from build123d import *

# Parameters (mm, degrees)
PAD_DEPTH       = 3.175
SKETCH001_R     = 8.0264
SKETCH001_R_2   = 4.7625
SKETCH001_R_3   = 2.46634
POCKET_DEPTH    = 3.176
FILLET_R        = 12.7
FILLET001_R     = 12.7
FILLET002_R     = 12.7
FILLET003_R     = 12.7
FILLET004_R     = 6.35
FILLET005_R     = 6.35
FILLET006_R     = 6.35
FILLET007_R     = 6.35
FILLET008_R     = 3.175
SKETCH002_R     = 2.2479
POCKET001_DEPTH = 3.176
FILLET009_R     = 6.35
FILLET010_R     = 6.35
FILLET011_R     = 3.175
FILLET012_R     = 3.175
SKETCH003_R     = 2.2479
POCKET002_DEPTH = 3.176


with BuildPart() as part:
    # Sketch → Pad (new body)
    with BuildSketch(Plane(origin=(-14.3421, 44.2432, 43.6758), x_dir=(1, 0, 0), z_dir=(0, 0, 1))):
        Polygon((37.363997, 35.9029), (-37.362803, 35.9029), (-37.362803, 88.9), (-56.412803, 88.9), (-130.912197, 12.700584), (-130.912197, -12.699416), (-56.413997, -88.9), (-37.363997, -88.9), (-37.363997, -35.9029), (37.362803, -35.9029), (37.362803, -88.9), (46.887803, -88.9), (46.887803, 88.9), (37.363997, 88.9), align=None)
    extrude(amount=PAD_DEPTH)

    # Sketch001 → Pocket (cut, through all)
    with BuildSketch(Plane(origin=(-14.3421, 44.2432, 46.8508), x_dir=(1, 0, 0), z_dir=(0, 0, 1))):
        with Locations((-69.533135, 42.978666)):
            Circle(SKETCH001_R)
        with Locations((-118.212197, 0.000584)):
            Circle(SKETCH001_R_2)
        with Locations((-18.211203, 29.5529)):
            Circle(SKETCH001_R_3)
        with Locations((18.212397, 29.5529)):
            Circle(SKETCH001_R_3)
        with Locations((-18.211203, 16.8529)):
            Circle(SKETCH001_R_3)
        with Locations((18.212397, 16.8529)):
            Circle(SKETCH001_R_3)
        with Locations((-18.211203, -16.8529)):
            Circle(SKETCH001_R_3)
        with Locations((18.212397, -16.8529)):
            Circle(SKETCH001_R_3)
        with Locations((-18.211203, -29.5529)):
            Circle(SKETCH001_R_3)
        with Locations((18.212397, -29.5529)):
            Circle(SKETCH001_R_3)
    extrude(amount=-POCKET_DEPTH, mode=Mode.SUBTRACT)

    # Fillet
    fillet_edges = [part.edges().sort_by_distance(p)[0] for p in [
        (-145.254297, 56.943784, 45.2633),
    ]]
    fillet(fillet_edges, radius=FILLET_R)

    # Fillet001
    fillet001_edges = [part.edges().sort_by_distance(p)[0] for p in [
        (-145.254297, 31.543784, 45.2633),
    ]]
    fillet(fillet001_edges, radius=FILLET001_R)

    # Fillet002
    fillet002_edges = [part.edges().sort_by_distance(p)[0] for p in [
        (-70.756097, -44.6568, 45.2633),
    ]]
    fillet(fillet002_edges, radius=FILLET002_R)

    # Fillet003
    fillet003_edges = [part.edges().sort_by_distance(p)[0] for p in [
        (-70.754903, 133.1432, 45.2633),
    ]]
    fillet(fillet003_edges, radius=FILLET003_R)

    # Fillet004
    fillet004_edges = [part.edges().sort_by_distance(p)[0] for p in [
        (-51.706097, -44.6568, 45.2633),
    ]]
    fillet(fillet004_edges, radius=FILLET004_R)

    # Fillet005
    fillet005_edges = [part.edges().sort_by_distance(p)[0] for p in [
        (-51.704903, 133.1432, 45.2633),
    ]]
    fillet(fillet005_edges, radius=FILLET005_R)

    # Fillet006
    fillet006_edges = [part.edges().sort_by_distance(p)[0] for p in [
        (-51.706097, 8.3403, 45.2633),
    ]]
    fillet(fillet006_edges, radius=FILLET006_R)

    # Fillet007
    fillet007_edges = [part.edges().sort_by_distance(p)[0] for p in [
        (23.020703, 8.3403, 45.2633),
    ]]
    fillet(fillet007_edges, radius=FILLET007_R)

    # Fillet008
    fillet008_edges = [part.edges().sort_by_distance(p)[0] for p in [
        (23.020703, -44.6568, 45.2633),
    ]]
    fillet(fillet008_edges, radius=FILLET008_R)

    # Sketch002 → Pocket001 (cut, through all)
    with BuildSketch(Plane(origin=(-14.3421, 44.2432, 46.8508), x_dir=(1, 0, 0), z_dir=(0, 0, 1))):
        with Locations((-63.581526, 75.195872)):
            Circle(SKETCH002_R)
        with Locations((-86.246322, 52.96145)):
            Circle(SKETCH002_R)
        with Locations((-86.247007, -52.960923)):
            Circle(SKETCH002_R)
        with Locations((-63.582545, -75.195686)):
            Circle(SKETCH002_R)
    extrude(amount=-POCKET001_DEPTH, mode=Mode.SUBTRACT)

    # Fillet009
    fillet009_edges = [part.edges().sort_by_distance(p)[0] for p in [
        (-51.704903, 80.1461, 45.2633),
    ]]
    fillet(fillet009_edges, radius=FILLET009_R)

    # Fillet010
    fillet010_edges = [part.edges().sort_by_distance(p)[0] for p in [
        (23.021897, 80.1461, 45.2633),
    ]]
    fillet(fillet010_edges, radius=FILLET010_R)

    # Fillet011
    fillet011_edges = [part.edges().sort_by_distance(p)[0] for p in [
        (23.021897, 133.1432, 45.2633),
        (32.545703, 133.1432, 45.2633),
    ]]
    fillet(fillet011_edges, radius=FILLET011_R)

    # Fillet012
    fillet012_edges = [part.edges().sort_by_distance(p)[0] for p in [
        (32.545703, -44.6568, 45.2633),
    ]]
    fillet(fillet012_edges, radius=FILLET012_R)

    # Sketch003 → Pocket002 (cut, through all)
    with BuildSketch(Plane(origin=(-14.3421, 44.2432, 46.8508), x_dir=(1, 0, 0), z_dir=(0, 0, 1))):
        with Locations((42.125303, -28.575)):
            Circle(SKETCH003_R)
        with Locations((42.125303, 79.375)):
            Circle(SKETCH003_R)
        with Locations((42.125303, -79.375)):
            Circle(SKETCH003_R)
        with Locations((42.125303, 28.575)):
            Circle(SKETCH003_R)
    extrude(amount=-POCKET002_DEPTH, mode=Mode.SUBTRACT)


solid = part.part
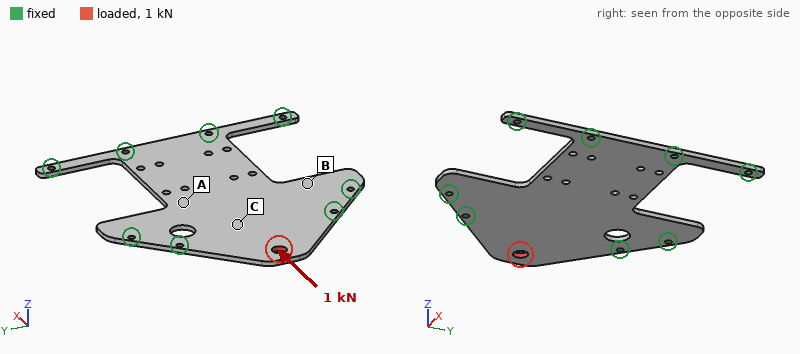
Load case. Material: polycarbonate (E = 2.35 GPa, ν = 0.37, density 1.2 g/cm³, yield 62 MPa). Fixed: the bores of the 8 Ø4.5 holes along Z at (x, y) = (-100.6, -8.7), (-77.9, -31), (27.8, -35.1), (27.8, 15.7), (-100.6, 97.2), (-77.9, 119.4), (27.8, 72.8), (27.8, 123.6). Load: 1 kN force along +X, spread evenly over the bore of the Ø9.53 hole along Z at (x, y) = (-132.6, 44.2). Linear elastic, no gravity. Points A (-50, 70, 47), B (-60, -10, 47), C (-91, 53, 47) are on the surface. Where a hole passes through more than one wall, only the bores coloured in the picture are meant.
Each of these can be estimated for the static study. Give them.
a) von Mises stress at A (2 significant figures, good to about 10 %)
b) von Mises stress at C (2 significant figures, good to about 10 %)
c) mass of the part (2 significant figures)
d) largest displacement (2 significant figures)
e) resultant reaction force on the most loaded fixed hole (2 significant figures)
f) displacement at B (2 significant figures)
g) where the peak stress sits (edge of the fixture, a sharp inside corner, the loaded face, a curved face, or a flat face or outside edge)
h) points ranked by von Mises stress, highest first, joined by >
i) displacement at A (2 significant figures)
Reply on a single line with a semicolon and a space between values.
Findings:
2.5 MPa; 3.9 MPa; 67 g; 0.28 mm; 330 N; 0.049 mm; the loaded face; C > A > B; 0.074 mm
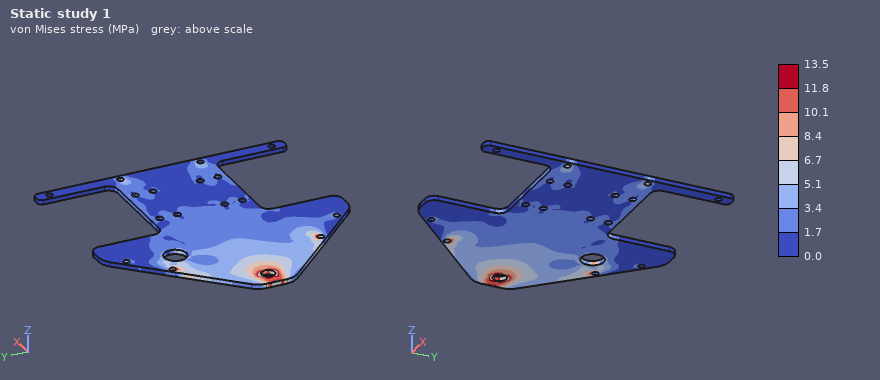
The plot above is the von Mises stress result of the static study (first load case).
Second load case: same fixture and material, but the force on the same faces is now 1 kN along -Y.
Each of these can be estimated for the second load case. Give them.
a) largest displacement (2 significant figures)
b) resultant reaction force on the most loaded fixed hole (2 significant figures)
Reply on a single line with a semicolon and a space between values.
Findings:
0.32 mm; 500 N
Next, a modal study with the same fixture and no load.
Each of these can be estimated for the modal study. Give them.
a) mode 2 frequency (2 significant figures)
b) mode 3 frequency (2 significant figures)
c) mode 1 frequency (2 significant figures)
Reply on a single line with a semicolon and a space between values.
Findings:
260 Hz; 500 Hz; 250 Hz
